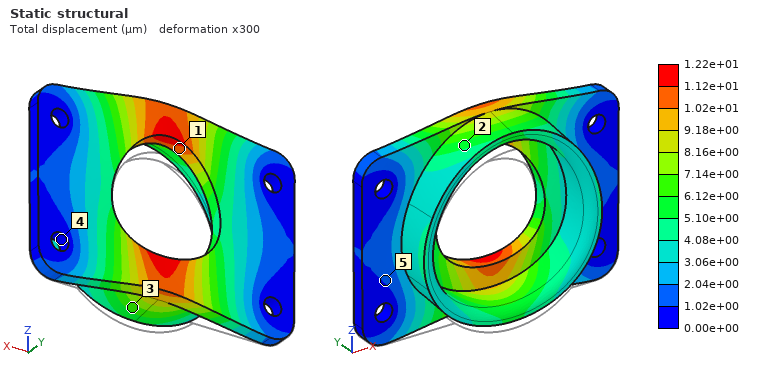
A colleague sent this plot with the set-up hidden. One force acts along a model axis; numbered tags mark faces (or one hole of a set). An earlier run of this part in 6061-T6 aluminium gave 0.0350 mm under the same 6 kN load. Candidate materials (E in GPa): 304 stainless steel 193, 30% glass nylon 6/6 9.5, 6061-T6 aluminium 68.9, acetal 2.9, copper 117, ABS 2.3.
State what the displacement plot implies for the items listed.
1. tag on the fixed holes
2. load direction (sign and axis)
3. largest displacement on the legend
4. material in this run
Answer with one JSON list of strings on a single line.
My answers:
["4", "+Z", "1.22e+01 µm", "304 stainless steel"]
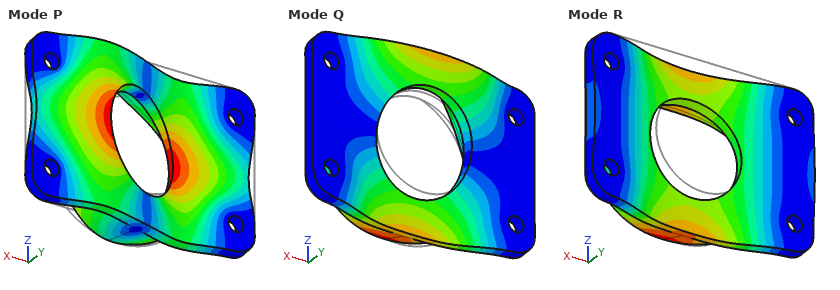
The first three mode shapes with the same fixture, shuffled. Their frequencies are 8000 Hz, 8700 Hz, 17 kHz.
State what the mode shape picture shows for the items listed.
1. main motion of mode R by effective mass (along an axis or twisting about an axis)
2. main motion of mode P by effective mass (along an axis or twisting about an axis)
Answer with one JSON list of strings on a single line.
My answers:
["along Y", "twisting about Z"]
